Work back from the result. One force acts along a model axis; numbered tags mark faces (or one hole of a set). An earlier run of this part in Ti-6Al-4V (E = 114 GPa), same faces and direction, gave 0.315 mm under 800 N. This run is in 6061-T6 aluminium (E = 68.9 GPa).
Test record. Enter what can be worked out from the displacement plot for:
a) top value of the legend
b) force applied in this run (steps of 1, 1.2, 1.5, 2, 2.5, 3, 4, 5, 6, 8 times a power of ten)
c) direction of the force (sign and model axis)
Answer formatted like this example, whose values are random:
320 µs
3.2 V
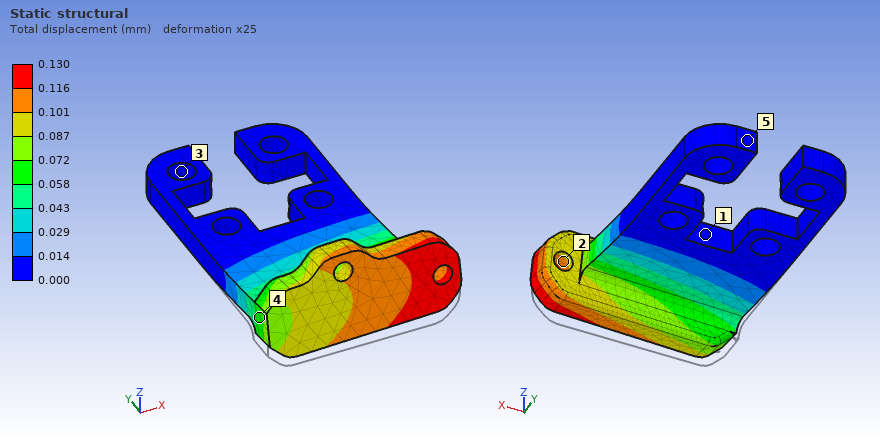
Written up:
0.130 mm
200 N
+Z
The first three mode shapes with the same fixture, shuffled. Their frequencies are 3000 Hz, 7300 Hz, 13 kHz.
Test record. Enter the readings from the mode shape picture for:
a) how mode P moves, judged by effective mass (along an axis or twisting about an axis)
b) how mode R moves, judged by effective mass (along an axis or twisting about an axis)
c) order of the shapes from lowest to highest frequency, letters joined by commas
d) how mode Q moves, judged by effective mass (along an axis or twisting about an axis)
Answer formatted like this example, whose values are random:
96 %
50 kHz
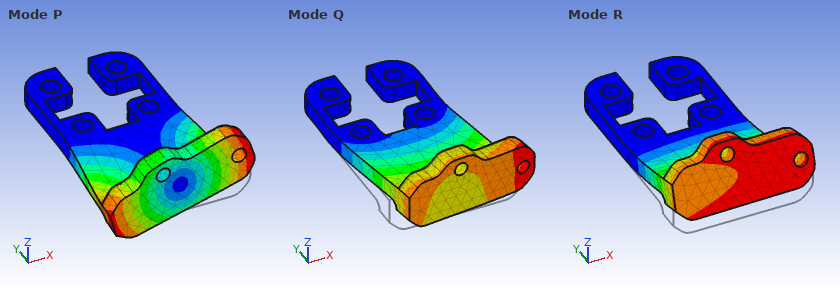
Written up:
twisting about Y
along Z
R, P, Q
along X
